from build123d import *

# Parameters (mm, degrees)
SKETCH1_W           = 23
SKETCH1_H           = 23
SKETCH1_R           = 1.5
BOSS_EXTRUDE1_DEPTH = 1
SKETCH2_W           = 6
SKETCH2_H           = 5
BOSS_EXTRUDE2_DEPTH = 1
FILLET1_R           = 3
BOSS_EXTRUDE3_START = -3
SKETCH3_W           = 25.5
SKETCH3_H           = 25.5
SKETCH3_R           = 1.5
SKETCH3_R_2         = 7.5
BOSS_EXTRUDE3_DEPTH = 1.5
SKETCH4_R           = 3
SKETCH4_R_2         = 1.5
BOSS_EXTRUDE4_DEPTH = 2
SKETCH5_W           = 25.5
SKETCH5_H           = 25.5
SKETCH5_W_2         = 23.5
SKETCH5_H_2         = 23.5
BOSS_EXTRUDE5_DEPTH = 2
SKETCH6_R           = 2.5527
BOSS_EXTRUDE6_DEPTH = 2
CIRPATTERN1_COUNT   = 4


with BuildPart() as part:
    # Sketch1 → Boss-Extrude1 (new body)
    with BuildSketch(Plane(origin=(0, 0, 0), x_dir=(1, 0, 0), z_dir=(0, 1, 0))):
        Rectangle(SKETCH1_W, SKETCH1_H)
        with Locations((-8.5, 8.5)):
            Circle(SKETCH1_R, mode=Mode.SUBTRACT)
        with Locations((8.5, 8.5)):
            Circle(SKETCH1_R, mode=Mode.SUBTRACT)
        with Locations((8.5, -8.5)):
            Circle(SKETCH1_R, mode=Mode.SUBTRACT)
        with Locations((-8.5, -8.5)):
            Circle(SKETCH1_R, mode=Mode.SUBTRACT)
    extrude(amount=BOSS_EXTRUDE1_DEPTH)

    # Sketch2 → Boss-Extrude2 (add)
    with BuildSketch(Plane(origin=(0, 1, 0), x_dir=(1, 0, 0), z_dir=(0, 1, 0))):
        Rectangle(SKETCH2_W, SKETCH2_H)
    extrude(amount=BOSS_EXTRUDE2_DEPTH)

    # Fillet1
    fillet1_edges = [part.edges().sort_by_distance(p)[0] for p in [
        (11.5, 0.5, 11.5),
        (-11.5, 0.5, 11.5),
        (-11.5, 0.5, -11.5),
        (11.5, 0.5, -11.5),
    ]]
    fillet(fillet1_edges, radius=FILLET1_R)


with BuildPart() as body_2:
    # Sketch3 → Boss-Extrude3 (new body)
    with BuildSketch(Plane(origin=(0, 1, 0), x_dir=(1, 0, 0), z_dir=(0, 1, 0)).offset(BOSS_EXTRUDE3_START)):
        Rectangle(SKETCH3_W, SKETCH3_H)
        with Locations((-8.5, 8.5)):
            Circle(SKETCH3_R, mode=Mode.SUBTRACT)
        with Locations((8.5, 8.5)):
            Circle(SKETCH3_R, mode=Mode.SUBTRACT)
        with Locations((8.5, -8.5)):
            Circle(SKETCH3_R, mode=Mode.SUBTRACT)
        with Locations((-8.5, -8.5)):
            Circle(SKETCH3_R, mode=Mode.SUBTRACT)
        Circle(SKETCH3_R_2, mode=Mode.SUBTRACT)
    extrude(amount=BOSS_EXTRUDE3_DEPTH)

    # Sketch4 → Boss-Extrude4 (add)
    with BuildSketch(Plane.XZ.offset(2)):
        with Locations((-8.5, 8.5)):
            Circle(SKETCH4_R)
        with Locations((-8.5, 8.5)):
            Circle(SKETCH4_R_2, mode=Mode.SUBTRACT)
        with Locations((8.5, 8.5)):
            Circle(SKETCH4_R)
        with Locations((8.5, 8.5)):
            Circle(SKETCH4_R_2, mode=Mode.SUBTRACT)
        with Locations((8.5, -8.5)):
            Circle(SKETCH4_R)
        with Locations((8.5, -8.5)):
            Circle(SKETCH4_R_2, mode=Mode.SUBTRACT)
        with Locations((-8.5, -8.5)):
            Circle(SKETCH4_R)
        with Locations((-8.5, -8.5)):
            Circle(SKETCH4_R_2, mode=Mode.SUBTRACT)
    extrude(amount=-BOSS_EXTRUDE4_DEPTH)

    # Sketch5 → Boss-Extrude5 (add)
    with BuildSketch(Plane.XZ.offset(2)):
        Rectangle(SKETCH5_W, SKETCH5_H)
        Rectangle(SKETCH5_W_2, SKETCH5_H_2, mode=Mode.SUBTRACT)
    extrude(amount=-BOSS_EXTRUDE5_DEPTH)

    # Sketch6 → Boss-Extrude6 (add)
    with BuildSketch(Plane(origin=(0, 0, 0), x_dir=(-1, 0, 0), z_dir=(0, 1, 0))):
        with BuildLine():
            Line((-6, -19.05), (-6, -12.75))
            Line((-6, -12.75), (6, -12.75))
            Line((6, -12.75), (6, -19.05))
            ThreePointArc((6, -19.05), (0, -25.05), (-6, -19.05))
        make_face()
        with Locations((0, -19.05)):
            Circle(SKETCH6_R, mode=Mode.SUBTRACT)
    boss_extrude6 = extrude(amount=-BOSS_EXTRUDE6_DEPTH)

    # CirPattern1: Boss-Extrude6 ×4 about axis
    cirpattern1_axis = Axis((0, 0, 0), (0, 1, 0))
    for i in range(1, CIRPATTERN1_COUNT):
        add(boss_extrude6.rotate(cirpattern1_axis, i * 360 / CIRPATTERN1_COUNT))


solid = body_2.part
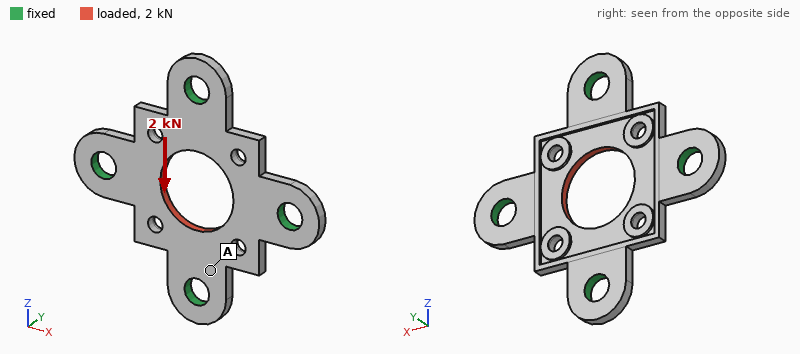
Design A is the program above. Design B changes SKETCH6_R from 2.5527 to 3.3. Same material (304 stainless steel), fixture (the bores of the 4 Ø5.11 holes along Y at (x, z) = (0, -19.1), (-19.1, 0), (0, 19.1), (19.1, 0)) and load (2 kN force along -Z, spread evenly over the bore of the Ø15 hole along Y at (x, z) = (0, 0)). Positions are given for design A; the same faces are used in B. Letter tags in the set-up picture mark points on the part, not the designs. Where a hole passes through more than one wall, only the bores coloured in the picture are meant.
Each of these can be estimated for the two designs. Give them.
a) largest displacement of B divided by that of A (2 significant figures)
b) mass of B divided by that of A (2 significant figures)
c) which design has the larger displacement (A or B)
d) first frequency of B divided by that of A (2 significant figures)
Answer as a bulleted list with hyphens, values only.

- 0.88
- 0.93
- A
- 1.2
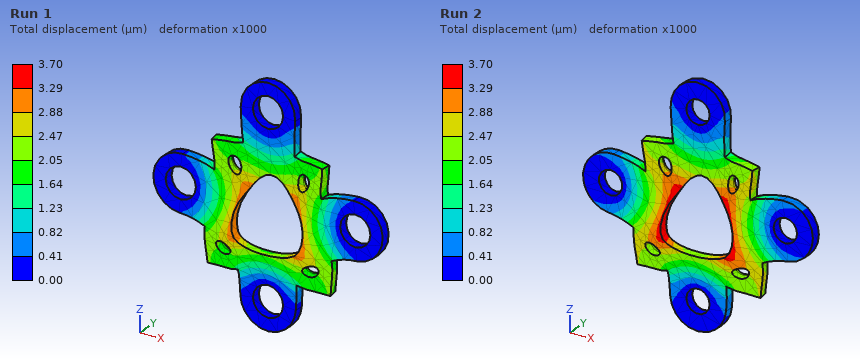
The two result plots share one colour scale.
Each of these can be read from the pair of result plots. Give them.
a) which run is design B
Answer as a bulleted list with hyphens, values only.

- Run 1
